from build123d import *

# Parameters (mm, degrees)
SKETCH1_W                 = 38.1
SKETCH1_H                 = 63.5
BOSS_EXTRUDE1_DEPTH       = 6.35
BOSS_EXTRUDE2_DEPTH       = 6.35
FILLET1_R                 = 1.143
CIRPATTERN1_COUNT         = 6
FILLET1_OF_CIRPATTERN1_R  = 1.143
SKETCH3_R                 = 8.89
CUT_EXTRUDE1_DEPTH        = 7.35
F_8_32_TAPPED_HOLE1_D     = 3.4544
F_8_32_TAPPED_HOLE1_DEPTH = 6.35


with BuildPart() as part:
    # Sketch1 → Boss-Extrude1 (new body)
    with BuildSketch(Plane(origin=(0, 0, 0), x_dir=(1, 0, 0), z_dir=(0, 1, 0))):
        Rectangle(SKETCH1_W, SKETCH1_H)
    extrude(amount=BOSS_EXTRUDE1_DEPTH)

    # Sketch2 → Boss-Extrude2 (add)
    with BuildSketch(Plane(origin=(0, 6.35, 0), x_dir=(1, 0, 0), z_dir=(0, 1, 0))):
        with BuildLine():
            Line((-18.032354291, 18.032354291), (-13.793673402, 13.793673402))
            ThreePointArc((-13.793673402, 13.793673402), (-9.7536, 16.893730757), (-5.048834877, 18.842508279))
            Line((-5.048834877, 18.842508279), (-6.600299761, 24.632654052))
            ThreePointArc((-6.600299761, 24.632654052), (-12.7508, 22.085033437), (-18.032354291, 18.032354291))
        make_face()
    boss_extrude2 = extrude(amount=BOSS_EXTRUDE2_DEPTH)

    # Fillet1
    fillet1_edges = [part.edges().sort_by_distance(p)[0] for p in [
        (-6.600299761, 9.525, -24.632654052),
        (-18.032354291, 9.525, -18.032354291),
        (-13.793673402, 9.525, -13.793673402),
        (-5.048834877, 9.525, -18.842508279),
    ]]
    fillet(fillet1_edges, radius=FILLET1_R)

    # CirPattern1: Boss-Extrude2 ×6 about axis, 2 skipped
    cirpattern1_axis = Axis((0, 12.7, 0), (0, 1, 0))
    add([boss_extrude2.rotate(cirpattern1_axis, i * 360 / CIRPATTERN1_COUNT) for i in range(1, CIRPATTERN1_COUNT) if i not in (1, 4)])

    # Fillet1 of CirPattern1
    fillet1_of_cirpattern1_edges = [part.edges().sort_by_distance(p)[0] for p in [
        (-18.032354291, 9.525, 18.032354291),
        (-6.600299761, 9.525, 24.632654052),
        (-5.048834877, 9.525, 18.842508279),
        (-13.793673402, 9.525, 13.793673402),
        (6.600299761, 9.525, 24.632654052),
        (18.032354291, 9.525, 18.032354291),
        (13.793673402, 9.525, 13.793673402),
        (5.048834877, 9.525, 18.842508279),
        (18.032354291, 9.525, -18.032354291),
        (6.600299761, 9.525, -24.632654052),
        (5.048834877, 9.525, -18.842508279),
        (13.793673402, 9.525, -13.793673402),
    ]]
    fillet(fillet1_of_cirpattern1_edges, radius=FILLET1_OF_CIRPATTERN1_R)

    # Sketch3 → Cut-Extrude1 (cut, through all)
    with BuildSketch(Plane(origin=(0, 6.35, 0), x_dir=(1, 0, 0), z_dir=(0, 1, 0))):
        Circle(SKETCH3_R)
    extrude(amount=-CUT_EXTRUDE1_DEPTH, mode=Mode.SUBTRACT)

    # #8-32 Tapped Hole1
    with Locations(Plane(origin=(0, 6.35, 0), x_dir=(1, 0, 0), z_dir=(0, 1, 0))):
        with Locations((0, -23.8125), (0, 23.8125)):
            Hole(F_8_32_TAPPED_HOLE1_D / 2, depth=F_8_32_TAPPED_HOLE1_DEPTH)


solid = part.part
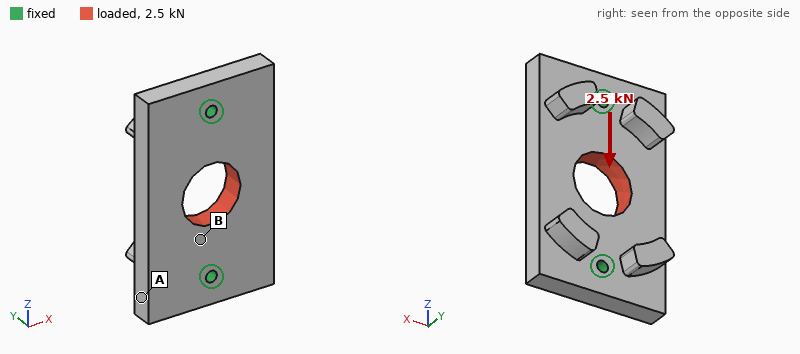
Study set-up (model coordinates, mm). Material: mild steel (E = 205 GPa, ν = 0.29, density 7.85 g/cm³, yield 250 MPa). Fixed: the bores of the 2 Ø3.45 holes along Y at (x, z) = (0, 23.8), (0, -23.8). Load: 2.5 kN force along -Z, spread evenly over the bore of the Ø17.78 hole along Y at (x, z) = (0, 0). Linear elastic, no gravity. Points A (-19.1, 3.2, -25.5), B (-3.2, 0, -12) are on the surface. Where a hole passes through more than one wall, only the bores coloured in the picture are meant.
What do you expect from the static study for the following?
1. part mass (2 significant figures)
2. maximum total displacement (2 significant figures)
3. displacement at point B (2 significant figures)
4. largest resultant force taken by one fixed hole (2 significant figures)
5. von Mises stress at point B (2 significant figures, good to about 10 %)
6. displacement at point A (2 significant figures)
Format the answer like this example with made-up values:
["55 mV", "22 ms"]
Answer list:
["120 g", "1.3 µm", "0.77 µm", "1.3 kN", "11 MPa", "0.95 µm"]
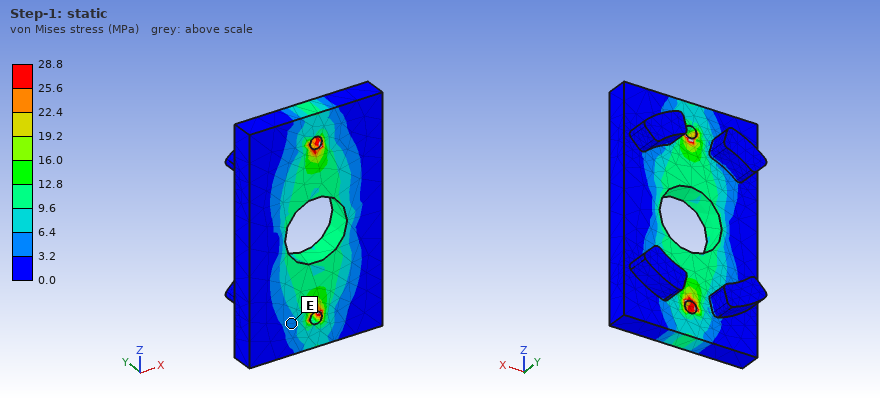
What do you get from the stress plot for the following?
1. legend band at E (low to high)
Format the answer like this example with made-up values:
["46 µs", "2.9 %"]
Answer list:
["3.2 to 6.4 MPa"]
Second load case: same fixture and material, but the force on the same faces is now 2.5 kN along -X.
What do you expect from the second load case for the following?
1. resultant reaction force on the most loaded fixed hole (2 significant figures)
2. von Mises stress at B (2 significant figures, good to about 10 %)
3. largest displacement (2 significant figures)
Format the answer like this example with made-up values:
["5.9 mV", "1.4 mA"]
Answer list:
["1.3 kN", "13 MPa", "2.7 µm"]
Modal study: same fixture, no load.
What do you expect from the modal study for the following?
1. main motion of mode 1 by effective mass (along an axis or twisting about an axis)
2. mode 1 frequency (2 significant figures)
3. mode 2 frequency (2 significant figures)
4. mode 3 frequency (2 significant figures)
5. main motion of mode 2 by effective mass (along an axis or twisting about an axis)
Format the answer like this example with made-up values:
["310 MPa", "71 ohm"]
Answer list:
["twisting about Z", "7200 Hz", "8800 Hz", "12 kHz", "along Y"]
